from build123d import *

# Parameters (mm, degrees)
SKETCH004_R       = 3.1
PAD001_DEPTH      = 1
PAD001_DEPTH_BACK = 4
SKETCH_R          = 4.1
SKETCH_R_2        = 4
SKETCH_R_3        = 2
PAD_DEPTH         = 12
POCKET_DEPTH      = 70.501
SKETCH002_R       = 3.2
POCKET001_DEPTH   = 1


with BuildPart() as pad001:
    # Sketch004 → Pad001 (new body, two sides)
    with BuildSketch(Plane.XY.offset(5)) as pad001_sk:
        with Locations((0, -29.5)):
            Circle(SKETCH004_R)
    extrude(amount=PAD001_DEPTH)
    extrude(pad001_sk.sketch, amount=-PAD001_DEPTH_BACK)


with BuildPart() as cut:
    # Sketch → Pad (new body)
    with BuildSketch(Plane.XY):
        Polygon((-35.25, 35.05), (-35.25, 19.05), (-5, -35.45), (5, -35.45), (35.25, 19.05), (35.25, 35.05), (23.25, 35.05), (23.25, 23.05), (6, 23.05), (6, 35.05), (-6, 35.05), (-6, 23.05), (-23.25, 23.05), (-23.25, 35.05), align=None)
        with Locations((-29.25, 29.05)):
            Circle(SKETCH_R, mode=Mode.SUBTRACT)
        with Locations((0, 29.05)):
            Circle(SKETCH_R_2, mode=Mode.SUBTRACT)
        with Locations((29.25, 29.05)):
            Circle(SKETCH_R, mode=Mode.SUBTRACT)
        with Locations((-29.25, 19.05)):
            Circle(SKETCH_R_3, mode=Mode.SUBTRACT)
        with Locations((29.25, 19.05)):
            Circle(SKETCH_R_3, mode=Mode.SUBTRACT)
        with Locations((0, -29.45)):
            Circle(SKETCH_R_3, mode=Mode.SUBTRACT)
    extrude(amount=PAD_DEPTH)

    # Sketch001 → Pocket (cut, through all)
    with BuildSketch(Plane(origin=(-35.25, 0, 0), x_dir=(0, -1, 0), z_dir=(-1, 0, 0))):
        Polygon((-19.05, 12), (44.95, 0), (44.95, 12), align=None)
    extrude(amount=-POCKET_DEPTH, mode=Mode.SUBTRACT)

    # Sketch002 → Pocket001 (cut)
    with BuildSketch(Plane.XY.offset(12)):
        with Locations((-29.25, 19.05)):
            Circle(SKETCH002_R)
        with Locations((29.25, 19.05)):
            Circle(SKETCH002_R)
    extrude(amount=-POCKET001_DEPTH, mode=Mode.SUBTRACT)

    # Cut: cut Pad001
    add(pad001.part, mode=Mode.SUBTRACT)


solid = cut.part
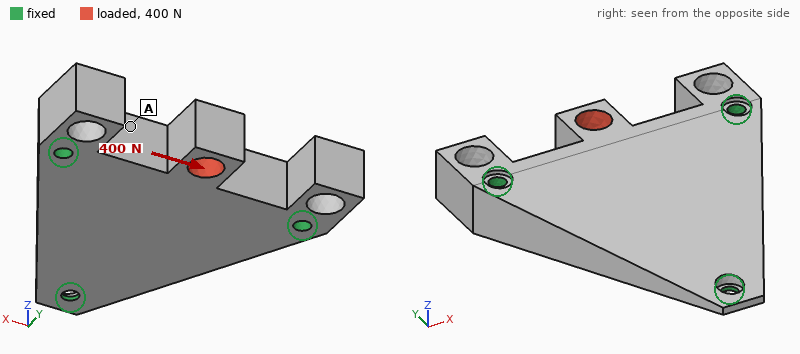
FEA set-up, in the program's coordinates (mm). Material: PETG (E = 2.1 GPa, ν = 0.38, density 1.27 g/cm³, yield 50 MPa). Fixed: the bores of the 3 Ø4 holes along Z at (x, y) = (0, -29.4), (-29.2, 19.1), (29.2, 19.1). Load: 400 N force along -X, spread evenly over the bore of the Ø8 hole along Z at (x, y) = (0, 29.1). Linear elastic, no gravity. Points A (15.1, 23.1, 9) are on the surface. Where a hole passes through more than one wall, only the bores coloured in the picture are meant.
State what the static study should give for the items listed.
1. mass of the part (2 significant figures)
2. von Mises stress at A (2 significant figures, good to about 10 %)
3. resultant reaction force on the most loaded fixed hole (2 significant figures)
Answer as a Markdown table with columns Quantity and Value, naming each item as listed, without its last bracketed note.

| Quantity | Value |
|---|---|
| mass of the part | 31 g |
| von Mises stress at A | 2.7 MPa |
| resultant reaction force on the most loaded fixed hole | 220 N |
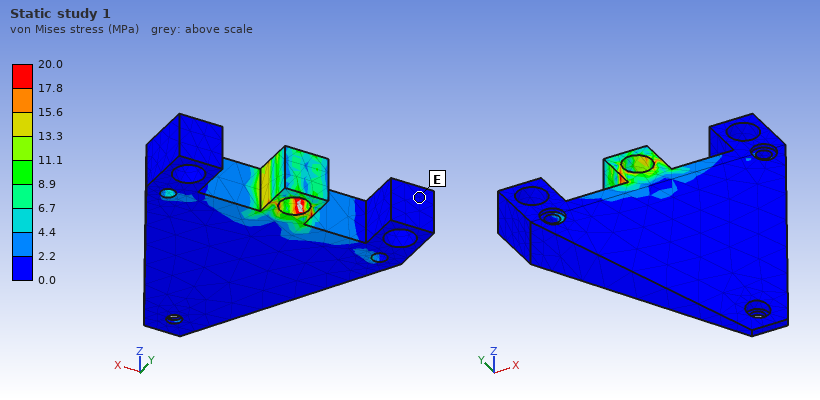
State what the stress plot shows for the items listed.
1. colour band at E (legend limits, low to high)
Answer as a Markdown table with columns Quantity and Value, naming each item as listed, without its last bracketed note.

| Quantity | Value |
|---|---|
| colour band at E | 0.0 to 2.2 MPa |
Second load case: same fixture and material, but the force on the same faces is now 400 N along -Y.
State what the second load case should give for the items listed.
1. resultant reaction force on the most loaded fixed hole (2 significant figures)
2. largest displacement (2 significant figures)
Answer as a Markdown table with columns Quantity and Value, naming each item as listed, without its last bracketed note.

| Quantity | Value |
|---|---|
| resultant reaction force on the most loaded fixed hole | 180 N |
| largest displacement | 95 µm |
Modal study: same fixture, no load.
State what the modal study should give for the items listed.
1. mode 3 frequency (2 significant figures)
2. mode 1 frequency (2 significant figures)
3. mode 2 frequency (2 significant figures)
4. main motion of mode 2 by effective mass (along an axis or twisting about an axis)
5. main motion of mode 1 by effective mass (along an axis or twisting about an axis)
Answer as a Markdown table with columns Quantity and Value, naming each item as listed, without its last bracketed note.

| Quantity | Value |
|---|---|
| mode 3 frequency | 3400 Hz |
| mode 1 frequency | 2000 Hz |
| mode 2 frequency | 2800 Hz |
| main motion of mode 2 by effective mass | along Z |
| main motion of mode 1 by effective mass | along Z |
